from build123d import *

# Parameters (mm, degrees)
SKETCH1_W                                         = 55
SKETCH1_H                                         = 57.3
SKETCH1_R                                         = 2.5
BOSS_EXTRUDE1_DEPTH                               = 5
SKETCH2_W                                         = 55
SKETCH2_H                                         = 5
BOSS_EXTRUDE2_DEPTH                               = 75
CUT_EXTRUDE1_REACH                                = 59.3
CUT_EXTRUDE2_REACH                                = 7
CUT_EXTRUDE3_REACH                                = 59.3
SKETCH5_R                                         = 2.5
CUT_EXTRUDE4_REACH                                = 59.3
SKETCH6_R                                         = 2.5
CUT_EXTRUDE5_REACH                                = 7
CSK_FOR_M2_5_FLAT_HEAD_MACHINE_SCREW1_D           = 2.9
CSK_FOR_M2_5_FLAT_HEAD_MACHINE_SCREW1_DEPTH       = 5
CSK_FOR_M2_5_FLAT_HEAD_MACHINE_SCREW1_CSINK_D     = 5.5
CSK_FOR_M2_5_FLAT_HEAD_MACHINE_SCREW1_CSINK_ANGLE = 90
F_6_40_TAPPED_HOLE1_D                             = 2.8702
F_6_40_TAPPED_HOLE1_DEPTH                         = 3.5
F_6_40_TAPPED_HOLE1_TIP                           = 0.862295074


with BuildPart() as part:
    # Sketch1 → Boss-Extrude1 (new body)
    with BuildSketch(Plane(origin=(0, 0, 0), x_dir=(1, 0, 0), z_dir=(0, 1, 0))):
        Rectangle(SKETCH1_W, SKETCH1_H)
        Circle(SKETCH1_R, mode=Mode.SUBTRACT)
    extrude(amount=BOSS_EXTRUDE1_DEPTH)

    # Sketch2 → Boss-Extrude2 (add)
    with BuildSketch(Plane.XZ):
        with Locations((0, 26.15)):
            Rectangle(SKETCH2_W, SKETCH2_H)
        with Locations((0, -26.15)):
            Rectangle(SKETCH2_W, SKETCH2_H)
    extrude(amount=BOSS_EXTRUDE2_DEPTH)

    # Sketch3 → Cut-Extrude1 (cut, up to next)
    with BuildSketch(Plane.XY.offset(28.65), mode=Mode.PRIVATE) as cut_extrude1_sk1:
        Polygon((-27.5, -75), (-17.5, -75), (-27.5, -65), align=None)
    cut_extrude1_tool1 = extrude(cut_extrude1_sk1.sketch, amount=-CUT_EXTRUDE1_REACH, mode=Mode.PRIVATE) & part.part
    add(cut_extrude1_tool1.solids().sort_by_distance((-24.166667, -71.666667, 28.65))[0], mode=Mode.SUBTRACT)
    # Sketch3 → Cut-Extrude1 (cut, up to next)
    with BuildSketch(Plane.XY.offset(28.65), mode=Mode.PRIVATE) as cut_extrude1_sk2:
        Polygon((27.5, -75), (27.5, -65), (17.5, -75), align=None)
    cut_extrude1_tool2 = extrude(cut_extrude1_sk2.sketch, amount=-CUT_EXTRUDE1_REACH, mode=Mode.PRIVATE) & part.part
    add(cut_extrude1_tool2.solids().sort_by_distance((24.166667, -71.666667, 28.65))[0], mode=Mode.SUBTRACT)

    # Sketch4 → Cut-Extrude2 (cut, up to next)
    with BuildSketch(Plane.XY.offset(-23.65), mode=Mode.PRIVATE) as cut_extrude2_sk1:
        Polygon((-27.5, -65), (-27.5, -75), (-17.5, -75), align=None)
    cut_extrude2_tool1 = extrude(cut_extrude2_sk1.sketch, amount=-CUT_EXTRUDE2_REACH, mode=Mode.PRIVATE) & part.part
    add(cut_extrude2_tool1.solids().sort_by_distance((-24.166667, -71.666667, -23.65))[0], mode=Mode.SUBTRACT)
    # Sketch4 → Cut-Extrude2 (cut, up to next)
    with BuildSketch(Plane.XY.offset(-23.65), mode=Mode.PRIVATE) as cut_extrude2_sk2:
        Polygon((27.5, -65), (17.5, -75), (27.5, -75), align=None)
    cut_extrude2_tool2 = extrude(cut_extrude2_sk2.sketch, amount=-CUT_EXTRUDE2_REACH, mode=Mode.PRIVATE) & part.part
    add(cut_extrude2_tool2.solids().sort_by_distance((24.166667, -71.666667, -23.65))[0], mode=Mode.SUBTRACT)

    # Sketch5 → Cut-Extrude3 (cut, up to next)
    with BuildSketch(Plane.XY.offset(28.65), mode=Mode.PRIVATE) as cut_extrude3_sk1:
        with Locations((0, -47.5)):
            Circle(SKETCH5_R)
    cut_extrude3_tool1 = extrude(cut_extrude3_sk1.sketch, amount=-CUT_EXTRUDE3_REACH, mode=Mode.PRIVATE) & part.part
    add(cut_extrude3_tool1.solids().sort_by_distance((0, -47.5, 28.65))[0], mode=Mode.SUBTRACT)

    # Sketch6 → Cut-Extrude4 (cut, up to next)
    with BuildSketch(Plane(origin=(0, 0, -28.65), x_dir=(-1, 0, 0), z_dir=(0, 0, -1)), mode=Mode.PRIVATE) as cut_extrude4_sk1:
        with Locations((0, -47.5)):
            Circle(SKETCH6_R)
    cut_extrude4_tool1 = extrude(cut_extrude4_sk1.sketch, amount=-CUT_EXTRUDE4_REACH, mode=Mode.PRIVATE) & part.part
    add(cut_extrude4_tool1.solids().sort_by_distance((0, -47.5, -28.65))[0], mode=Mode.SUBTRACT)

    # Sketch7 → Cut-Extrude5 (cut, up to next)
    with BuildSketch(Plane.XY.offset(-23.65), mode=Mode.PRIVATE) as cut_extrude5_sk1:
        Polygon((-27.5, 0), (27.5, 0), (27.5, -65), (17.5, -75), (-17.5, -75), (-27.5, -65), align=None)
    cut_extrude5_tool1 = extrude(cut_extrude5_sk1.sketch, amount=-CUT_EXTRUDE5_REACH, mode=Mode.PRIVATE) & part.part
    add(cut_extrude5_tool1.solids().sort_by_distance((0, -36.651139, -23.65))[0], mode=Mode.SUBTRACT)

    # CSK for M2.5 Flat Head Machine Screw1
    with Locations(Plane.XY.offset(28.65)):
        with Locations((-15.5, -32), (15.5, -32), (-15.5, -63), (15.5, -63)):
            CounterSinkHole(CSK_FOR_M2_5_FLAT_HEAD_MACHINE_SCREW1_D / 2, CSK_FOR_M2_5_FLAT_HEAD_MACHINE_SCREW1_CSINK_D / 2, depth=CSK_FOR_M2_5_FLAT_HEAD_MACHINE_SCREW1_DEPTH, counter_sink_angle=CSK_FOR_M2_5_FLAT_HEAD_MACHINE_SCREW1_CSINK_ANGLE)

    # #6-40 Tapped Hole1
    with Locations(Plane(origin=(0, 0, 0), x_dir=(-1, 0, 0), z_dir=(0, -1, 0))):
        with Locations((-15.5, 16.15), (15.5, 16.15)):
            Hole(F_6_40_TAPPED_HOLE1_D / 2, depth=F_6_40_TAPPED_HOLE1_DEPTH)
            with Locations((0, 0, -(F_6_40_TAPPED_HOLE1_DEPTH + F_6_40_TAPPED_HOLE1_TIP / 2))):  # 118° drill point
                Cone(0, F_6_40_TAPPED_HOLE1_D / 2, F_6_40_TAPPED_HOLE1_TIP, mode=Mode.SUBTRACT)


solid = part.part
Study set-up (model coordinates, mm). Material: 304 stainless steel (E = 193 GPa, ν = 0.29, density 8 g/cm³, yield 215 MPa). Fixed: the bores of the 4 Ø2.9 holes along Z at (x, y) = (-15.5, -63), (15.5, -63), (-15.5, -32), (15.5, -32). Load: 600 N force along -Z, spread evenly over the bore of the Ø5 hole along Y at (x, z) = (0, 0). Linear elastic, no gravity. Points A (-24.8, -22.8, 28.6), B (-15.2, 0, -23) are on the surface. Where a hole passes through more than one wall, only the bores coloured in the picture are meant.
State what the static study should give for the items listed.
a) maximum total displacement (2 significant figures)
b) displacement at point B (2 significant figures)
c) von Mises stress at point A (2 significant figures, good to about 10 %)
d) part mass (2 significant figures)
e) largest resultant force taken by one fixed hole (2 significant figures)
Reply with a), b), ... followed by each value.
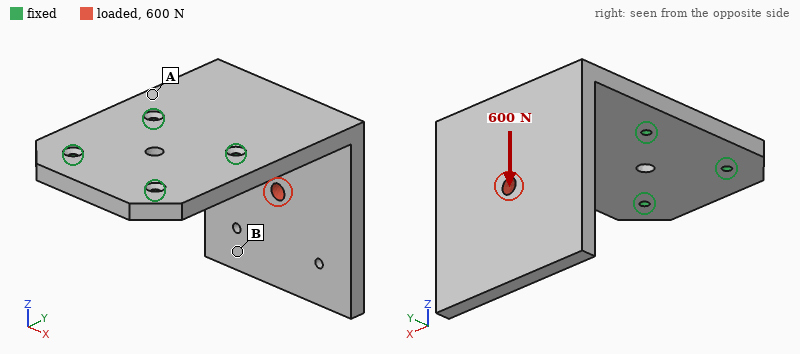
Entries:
a) 0.23 mm
b) 0.20 mm
c) 68 MPa
d) 280 g
e) 520 N
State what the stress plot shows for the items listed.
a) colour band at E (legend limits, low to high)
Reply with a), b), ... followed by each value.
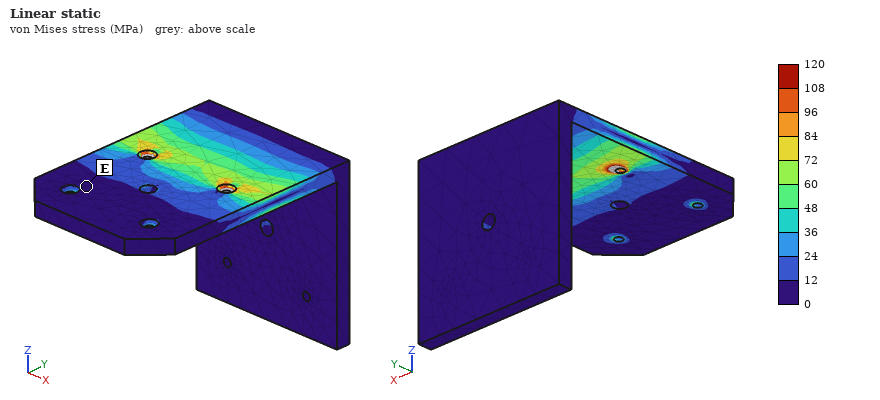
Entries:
a) 0 to 12 MPa
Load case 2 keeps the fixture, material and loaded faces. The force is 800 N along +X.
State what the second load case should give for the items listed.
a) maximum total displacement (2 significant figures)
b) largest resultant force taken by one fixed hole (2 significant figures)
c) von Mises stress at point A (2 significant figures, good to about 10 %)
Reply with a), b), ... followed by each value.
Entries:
a) 0.16 mm
b) 940 N
c) 47 MPa
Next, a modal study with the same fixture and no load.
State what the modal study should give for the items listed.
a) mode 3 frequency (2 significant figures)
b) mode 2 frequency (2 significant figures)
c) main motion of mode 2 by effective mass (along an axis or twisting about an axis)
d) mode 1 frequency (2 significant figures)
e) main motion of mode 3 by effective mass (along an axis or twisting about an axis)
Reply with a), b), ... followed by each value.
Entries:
a) 1800 Hz
b) 1100 Hz
c) along X
d) 620 Hz
e) along Z
